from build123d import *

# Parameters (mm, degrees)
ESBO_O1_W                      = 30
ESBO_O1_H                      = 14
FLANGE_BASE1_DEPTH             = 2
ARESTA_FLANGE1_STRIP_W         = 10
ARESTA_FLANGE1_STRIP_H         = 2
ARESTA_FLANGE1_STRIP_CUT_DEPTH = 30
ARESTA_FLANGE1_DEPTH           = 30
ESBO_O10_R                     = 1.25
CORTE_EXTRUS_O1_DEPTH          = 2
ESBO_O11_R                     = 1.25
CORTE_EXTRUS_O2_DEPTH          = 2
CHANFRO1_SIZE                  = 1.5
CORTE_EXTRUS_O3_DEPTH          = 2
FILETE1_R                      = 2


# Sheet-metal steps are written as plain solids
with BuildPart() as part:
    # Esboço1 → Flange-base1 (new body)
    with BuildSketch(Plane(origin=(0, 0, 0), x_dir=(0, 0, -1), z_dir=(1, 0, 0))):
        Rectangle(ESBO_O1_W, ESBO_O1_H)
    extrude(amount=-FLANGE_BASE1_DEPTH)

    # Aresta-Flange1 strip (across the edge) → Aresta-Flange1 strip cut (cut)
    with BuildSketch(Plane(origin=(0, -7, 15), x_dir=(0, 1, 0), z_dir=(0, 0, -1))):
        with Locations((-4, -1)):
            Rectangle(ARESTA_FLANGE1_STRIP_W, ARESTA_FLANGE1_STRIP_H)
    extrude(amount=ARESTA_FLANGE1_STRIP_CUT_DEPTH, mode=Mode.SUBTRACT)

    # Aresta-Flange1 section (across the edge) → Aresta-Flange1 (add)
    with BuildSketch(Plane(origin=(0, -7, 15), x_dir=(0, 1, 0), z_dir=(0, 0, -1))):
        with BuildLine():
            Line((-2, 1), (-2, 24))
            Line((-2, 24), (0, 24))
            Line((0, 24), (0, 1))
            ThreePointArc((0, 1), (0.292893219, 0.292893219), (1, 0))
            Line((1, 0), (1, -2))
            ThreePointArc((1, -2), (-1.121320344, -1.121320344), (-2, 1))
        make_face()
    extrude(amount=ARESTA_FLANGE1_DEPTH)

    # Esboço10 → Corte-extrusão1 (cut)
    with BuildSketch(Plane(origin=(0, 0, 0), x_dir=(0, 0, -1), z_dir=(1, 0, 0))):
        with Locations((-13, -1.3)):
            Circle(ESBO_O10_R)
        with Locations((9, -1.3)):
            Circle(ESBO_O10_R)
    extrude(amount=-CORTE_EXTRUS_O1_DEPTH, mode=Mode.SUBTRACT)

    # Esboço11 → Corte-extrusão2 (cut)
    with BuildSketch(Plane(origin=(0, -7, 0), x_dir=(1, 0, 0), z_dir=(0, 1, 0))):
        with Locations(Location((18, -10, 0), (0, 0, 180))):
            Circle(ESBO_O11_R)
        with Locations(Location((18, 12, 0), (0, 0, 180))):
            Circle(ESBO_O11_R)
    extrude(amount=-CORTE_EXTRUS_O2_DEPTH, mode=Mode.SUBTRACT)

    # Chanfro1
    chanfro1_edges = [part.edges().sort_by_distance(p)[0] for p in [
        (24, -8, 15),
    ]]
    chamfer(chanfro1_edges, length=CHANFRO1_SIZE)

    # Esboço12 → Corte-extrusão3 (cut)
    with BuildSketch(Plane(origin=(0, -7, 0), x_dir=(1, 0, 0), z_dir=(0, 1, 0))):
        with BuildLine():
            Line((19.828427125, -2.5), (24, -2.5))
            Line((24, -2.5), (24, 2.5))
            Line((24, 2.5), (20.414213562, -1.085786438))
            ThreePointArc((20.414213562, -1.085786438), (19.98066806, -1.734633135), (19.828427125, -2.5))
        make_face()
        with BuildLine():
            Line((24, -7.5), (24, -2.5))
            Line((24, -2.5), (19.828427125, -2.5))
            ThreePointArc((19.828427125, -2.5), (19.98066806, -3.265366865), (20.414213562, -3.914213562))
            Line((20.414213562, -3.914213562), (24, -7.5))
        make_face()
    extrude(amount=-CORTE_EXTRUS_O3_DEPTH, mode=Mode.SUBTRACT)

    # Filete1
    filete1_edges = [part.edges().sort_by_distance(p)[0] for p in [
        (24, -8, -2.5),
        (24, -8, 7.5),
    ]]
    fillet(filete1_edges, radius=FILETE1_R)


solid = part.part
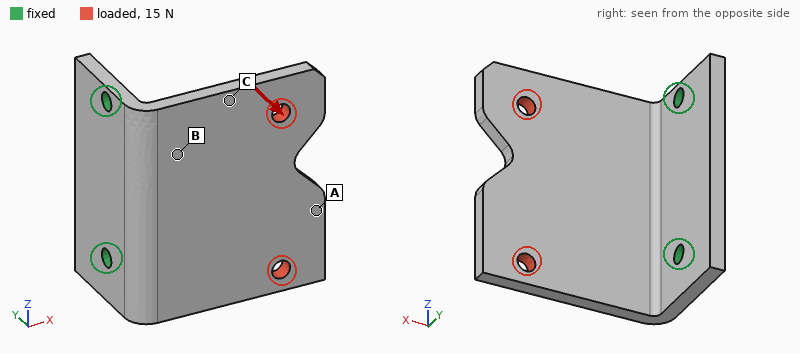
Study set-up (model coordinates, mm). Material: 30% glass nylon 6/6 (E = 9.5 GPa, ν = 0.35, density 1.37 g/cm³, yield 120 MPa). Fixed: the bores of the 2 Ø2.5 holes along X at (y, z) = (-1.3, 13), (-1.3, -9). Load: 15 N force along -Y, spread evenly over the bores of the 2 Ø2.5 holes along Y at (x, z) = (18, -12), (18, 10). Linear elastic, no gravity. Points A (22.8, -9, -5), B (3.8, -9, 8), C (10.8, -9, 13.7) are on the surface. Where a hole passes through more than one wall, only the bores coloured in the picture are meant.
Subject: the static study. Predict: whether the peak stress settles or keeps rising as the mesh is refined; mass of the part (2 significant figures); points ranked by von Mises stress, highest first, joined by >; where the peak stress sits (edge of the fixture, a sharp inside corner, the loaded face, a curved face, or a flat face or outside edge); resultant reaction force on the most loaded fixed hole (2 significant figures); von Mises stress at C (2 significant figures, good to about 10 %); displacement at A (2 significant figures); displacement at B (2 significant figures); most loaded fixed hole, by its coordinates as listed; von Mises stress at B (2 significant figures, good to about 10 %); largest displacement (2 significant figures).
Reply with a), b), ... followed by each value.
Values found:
a) keeps rising
b) 3.1 g
c) B > C > A
d) edge of the fixture
e) 9.6 N
f) 5.7 MPa
g) 0.45 mm
h) 0.077 mm
i) (-1.3, -9)
j) 9.1 MPa
k) 0.49 mm
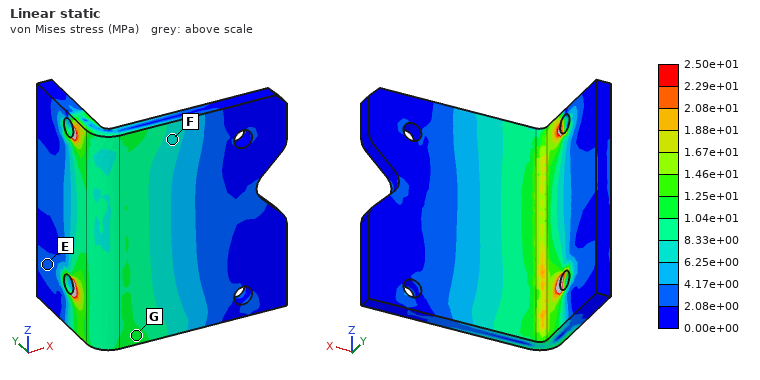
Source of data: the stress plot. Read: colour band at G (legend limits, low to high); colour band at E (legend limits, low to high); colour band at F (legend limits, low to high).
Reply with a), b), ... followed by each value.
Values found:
a) 1.04e+01 to 1.25e+01 MPa
b) 2.08e+00 to 4.17e+00 MPa
c) 6.25e+00 to 8.33e+00 MPa
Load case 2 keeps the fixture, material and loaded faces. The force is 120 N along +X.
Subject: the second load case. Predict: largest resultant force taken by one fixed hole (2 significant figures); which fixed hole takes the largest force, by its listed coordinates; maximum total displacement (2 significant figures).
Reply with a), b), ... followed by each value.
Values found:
a) 74 N
b) (-1.3, -9)
c) 0.42 mm
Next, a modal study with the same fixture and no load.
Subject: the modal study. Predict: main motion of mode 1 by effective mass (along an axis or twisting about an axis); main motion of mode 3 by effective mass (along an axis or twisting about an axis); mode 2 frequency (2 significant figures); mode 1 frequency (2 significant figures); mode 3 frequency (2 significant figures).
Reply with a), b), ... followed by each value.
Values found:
a) along Y
b) along Z
c) 2400 Hz
d) 1000 Hz
e) 3900 Hz
